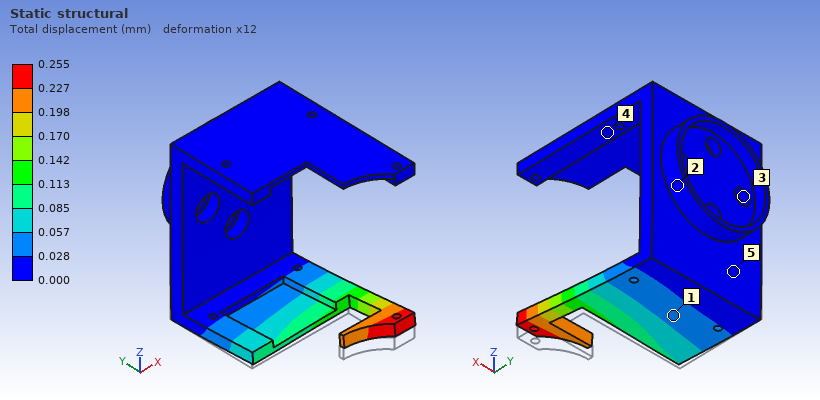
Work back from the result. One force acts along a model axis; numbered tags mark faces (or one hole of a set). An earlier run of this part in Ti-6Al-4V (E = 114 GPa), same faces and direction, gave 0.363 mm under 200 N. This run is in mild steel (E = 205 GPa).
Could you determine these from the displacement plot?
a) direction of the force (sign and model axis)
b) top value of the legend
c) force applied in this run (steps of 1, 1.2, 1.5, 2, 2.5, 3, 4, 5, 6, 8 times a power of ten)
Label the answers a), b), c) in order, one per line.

a) +Z
b) 0.255 mm
c) 250 N
